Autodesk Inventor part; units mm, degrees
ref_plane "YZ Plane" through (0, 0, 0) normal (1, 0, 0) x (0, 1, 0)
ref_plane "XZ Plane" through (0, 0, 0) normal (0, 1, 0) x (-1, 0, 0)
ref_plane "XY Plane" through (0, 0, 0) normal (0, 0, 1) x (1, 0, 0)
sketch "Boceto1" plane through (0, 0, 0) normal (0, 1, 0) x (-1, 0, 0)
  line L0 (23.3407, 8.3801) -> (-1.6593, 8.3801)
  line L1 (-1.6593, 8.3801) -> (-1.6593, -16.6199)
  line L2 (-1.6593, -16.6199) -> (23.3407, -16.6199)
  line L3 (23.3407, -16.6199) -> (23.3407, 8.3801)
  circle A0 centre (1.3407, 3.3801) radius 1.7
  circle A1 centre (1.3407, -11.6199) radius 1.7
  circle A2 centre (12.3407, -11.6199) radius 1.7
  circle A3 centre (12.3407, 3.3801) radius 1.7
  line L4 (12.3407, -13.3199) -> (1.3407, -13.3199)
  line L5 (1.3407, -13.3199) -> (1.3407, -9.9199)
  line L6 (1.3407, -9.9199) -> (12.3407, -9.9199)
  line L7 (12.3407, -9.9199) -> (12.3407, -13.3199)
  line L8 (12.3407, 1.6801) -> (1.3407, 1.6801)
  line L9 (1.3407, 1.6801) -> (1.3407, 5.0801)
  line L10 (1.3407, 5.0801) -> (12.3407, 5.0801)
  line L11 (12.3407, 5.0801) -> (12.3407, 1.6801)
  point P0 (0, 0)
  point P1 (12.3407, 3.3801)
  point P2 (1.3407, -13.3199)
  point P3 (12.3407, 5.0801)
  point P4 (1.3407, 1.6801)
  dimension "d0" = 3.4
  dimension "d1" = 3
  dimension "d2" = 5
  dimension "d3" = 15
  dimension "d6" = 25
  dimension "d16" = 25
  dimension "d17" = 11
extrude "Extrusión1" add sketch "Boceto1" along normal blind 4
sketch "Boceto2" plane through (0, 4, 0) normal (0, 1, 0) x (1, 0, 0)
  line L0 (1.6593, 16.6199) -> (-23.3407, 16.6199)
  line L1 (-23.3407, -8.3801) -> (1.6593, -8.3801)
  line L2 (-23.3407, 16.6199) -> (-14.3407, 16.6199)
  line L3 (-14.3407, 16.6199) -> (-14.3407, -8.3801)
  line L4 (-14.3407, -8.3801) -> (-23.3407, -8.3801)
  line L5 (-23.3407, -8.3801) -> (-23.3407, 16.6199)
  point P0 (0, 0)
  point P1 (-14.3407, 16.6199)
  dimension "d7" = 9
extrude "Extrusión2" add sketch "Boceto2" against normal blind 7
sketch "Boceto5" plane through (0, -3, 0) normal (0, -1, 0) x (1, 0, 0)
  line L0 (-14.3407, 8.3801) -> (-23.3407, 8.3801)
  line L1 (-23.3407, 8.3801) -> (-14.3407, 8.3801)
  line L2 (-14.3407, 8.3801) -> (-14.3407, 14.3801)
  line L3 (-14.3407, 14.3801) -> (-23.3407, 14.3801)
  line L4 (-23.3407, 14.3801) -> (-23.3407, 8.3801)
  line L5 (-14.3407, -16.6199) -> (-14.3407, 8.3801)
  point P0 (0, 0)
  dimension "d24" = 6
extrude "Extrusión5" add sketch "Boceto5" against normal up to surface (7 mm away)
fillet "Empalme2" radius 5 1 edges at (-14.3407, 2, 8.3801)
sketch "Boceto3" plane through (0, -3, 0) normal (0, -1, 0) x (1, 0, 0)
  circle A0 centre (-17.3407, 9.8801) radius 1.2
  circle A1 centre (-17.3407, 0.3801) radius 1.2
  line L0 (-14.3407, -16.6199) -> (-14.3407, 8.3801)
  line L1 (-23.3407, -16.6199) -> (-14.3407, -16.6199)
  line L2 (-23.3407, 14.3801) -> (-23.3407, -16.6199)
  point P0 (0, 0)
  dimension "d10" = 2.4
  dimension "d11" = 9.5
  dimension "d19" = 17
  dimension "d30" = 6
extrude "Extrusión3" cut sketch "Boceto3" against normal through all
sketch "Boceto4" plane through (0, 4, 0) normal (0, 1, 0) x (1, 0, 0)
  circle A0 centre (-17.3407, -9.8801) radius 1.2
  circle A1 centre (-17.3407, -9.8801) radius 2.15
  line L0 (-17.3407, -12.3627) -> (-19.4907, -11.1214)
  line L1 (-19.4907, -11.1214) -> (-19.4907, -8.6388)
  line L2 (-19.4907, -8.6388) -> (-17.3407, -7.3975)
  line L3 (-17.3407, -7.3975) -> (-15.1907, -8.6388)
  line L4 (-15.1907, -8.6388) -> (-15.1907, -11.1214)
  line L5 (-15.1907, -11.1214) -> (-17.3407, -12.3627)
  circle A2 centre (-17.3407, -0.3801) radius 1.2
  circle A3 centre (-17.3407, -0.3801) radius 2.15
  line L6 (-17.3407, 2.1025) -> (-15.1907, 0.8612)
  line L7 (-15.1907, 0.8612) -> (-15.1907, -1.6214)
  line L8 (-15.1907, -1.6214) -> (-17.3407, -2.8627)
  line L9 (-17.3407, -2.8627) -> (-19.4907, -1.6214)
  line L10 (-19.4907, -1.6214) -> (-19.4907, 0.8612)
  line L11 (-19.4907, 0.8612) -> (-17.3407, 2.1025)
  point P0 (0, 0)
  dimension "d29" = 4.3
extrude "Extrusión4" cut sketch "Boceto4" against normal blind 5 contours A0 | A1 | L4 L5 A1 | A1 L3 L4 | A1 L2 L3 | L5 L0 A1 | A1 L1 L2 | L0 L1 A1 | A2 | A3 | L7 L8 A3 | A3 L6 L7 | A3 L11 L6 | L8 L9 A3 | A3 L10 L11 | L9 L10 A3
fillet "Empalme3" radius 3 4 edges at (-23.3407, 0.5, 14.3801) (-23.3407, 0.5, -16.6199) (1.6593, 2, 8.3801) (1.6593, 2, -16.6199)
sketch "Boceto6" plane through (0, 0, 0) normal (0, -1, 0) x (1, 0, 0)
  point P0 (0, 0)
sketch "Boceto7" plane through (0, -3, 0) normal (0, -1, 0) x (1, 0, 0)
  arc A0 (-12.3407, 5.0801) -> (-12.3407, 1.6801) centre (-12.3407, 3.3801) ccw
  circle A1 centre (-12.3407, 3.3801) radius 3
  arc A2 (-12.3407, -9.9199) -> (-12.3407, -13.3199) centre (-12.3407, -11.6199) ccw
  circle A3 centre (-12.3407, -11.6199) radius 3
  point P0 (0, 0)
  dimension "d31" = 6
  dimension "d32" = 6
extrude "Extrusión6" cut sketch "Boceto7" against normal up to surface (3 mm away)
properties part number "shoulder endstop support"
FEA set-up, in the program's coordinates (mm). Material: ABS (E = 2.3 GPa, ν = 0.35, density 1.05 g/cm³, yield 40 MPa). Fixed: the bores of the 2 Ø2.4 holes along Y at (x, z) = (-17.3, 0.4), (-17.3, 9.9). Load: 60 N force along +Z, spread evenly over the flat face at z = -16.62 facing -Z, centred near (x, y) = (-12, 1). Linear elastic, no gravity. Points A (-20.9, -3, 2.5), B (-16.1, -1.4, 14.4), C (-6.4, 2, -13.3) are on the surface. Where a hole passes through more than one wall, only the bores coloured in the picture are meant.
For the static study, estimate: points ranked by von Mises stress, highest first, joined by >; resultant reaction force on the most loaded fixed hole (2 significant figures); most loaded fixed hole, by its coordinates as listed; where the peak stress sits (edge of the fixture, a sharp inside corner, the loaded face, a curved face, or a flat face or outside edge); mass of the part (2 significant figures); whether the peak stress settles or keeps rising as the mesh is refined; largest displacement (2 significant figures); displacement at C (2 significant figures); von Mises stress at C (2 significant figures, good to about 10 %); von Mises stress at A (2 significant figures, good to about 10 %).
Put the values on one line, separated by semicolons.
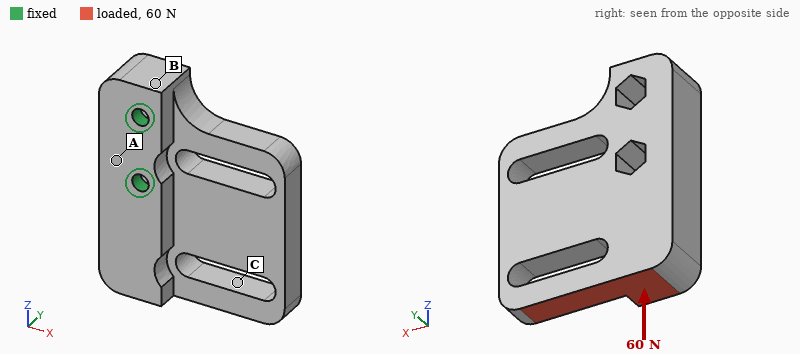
C > A > B; 52 N; (-17.3, 0.4); edge of the fixture; 3.1 g; keeps rising; 0.12 mm; 0.10 mm; 4.8 MPa; 2.2 MPa
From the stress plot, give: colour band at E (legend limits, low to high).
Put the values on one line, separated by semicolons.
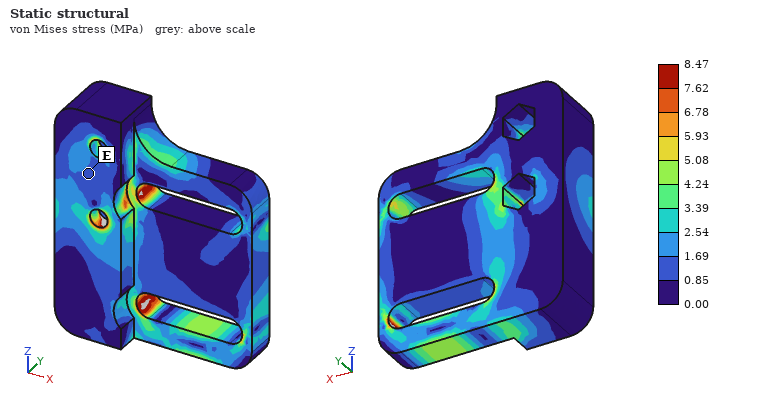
0.85 to 1.69 MPa
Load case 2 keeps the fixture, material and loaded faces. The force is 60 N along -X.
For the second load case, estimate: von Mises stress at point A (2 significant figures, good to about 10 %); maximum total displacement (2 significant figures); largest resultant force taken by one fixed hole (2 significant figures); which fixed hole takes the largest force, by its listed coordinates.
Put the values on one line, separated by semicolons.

9.3 MPa; 0.32 mm; 140 N; (-17.3, 0.4)
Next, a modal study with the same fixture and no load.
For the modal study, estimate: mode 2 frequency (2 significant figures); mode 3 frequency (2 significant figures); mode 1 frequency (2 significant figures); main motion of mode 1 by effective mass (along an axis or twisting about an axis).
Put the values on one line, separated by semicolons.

2400 Hz; 3000 Hz; 1500 Hz; along Y
